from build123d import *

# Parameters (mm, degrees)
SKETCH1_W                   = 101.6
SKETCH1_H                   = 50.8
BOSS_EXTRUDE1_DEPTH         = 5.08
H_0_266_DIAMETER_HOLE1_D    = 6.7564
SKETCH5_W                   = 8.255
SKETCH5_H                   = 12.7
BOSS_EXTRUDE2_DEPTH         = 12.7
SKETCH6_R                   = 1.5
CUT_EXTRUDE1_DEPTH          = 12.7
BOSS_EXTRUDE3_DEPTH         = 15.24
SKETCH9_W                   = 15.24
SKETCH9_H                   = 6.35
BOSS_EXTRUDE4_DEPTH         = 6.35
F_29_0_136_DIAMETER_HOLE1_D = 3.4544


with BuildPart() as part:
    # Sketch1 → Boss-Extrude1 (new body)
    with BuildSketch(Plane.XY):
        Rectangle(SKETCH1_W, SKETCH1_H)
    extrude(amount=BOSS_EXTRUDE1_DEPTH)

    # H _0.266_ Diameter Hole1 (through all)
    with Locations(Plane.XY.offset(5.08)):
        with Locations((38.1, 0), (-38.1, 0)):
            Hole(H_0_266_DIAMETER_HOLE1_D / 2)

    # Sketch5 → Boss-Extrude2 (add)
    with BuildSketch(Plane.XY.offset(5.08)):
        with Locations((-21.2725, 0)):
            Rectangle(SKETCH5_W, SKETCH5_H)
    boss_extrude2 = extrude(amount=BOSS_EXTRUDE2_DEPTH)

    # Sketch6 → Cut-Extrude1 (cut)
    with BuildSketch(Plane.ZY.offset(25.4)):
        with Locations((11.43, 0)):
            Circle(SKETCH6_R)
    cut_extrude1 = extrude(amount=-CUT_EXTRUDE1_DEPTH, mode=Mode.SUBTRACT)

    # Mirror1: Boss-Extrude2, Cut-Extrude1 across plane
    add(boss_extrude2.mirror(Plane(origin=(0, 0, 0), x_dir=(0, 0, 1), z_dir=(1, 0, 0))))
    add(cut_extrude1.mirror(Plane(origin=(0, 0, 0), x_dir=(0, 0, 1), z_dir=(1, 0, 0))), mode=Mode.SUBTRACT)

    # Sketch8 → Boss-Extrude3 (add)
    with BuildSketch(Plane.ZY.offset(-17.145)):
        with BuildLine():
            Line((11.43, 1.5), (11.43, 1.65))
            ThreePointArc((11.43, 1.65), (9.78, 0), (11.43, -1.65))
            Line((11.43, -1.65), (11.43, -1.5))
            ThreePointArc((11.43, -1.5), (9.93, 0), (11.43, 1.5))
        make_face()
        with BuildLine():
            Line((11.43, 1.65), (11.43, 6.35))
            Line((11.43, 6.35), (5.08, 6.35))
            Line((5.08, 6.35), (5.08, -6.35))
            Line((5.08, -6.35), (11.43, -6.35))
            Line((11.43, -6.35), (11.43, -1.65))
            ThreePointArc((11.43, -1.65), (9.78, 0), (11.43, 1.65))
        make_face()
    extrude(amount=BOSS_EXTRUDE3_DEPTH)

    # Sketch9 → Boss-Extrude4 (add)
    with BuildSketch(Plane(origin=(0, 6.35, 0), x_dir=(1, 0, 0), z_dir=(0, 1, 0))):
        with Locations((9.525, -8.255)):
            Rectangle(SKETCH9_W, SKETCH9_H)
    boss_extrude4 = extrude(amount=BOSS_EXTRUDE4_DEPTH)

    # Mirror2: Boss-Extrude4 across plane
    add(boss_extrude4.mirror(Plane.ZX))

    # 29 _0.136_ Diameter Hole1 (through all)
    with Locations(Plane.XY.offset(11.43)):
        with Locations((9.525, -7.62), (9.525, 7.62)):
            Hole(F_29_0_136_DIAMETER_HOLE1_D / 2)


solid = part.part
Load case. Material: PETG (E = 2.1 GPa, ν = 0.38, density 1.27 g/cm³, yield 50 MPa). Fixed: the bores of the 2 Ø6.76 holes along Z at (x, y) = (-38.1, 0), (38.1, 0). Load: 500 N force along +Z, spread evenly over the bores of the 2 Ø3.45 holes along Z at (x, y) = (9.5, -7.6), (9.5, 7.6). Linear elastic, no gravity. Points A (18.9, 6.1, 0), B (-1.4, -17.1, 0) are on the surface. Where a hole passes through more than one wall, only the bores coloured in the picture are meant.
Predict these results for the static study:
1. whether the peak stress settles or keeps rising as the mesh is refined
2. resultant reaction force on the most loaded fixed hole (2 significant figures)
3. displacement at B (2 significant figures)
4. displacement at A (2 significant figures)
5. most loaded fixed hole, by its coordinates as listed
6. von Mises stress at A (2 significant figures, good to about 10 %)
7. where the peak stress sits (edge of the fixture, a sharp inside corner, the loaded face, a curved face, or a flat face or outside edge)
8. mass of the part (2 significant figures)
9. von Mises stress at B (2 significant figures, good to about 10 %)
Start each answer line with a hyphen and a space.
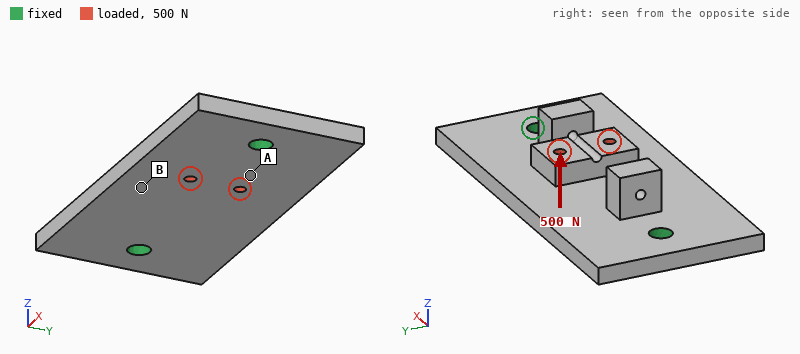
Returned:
- keeps rising
- 340 N
- 0.79 mm
- 0.48 mm
- (38.1, 0)
- 4.1 MPa
- edge of the fixture
- 39 g
- 12 MPa
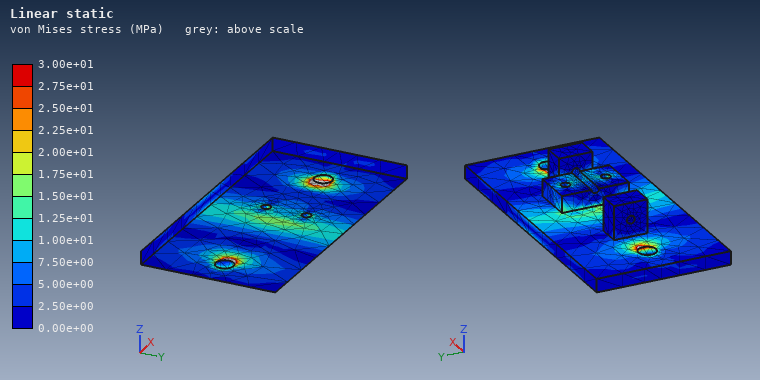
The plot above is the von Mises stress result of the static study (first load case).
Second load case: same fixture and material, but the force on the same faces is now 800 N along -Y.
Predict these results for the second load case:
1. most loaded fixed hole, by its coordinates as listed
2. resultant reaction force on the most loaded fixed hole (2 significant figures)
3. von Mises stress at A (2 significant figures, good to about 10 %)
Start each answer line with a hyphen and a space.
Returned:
- (38.1, 0)
- 510 N
- 2.5 MPa
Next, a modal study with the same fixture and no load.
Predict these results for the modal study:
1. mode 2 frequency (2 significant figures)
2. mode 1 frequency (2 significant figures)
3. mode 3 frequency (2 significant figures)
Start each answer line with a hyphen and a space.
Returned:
- 970 Hz
- 950 Hz
- 1800 Hz
